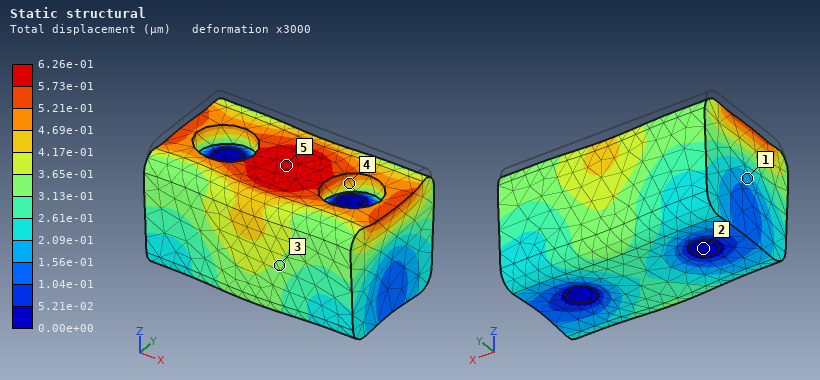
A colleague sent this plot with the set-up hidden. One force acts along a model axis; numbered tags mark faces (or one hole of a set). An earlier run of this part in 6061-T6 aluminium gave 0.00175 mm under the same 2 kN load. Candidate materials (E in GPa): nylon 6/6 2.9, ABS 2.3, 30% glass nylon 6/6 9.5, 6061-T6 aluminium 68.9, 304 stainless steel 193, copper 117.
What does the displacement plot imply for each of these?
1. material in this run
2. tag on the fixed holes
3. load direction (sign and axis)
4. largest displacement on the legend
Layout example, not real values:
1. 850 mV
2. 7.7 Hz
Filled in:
1. 304 stainless steel
2. 2
3. -Z
4. 6.26e-01 µm
